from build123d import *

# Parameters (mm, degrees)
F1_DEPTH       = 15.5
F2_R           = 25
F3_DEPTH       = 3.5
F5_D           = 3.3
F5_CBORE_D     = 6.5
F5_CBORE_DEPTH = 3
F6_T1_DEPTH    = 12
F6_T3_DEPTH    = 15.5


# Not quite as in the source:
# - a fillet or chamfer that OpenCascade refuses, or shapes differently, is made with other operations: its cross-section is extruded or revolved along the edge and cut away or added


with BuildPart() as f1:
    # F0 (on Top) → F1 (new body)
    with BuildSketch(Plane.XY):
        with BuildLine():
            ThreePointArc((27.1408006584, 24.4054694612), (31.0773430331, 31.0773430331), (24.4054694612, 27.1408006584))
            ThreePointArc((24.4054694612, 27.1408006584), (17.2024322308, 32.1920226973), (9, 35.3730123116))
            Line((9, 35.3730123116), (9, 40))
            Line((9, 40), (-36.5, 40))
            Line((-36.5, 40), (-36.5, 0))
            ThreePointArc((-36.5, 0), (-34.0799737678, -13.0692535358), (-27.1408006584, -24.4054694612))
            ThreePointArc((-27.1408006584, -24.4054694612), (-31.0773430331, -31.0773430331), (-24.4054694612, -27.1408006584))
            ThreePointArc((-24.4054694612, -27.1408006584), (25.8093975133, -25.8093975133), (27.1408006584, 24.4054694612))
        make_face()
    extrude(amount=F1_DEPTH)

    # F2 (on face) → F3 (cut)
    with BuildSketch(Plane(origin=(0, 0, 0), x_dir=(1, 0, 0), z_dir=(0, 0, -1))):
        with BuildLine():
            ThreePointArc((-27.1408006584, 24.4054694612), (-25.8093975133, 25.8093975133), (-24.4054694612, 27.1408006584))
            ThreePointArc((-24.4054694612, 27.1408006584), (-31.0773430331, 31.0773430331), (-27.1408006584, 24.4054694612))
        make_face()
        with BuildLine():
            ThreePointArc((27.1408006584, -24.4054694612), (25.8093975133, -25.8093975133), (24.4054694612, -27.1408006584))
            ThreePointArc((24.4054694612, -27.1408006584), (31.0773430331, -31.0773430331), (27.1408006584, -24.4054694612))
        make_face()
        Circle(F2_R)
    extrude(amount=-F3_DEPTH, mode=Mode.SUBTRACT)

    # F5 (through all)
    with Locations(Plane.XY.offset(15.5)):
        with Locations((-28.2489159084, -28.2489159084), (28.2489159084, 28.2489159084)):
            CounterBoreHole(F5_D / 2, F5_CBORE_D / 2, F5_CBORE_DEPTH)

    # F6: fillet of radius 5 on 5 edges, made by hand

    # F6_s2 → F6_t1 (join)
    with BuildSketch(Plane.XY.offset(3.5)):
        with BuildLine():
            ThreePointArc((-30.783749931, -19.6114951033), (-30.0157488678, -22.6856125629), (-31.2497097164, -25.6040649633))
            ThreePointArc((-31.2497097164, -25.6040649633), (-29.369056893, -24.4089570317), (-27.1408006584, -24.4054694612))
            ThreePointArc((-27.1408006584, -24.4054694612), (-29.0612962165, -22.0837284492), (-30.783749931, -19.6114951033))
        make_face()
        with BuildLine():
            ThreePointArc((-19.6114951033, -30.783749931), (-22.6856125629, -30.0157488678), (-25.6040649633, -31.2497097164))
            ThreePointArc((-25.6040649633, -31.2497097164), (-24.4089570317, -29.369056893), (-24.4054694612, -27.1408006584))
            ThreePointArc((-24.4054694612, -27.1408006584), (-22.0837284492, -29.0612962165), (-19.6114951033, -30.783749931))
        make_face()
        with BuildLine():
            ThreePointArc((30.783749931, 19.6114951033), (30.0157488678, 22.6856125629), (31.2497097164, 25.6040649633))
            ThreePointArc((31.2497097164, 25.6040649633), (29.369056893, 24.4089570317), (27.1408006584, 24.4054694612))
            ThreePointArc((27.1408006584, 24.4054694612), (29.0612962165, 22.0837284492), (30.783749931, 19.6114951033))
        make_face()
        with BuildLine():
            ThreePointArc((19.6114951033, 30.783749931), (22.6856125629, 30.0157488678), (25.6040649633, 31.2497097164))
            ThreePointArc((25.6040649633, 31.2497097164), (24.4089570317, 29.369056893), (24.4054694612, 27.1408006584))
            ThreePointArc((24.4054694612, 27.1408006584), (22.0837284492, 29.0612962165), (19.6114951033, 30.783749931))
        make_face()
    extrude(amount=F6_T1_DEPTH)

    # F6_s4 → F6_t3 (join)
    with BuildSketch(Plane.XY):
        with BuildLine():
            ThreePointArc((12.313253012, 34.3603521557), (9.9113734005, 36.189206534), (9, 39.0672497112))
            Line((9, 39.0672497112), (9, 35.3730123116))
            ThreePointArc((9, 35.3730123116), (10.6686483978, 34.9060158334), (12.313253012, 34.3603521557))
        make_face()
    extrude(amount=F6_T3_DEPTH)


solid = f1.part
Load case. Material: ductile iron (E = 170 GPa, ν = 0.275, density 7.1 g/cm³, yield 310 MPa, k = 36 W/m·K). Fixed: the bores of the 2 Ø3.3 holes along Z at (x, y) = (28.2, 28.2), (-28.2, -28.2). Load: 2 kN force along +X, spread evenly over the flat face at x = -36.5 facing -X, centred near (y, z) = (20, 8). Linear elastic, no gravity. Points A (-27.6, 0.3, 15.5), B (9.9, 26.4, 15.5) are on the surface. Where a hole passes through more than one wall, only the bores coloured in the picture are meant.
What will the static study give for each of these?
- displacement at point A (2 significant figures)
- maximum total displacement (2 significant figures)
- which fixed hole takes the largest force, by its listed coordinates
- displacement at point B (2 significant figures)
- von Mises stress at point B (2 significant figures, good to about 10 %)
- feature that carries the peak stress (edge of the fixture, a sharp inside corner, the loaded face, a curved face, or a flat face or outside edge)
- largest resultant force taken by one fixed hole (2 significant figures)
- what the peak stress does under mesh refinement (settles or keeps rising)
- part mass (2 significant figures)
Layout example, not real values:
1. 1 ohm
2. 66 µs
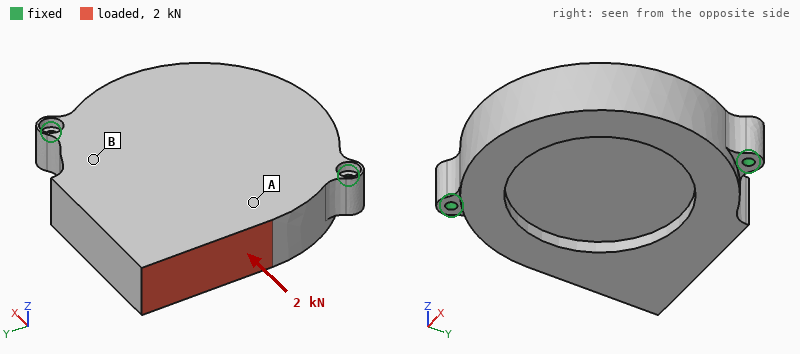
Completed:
1. 1.5 µm
2. 3.4 µm
3. (28.2, 28.2)
4. 1.4 µm
5. 5.5 MPa
6. edge of the fixture
7. 1.5 kN
8. keeps rising
9. 470 g
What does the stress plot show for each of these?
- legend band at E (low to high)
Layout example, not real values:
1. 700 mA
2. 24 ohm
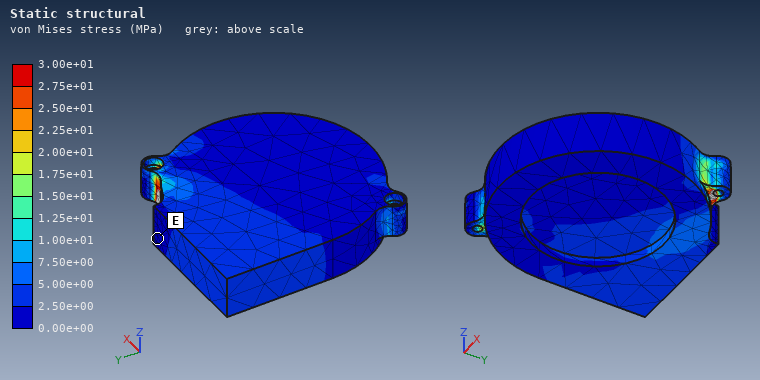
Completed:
1. 0.00e+00 to 2.50e+00 MPa
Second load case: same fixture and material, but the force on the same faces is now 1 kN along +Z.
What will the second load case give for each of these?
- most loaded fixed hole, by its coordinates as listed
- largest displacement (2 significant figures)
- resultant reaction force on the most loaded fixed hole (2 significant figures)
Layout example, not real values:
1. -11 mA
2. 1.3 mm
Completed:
1. (-28.2, -28.2)
2. 87 µm
3. 690 N
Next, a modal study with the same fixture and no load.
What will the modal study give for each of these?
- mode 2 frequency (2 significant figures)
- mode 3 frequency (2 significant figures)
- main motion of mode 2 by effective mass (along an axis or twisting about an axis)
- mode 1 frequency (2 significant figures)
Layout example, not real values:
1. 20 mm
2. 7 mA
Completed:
1. 4000 Hz
2. 8600 Hz
3. along Z
4. 1800 Hz
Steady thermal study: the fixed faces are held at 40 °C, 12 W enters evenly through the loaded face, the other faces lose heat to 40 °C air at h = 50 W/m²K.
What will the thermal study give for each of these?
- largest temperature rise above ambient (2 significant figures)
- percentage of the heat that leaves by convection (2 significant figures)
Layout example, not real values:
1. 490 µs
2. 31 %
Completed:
1. 24 K
2. 49 %
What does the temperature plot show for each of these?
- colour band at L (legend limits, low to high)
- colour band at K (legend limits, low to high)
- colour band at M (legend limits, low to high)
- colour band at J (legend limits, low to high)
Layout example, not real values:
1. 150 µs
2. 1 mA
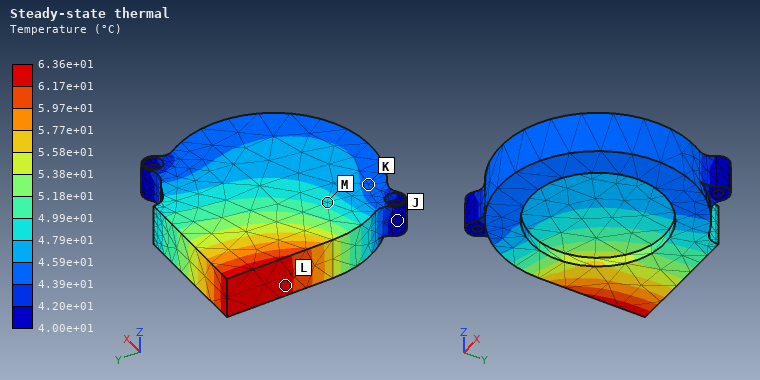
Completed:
1. 6.17e+01 to 6.36e+01 °C
2. 4.39e+01 to 4.59e+01 °C
3. 4.79e+01 to 4.99e+01 °C
4. 4.00e+01 to 4.20e+01 °C
